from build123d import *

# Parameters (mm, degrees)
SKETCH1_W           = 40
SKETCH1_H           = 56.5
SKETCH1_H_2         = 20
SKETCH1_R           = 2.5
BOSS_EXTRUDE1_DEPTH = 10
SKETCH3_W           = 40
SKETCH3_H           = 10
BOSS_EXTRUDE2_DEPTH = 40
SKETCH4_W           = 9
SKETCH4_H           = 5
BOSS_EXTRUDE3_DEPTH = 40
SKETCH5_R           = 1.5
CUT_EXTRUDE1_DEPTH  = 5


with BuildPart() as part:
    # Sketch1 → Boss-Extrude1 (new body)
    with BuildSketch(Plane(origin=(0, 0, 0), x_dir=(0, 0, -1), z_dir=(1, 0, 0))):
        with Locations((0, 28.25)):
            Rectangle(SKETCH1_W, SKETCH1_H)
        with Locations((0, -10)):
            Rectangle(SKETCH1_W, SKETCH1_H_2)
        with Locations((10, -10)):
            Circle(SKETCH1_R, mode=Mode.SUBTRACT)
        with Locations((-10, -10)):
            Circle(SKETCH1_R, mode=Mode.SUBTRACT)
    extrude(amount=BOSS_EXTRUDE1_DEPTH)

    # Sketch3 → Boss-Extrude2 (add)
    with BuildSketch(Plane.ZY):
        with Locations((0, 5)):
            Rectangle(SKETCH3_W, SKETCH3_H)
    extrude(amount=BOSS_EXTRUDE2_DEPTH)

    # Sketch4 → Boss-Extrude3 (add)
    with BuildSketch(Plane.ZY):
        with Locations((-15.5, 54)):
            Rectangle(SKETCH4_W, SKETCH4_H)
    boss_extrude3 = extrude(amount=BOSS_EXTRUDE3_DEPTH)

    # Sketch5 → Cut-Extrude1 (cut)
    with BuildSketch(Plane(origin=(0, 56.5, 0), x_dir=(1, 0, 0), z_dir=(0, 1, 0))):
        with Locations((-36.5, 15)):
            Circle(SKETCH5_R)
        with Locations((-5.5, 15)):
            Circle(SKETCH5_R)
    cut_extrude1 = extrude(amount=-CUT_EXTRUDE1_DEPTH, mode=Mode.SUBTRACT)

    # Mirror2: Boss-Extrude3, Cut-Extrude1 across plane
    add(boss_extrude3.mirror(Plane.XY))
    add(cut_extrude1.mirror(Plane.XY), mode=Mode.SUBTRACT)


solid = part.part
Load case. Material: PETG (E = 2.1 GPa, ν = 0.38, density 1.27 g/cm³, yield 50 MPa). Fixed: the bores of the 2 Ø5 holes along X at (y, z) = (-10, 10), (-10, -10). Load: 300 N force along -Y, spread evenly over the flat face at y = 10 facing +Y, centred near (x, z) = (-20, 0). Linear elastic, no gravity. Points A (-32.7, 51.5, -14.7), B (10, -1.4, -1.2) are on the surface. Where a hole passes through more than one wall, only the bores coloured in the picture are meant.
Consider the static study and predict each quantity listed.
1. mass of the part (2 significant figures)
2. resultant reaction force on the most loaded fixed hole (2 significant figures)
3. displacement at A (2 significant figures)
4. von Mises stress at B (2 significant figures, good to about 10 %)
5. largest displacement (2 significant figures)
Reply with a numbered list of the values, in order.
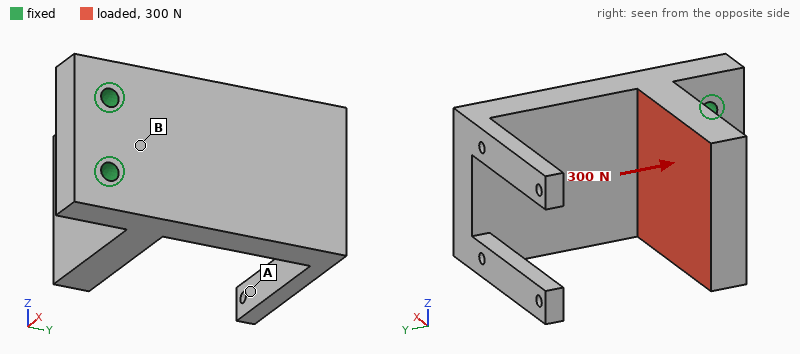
1. 63 g
2. 160 N
3. 0.96 mm
4. 8.4 MPa
5. 1.1 mm
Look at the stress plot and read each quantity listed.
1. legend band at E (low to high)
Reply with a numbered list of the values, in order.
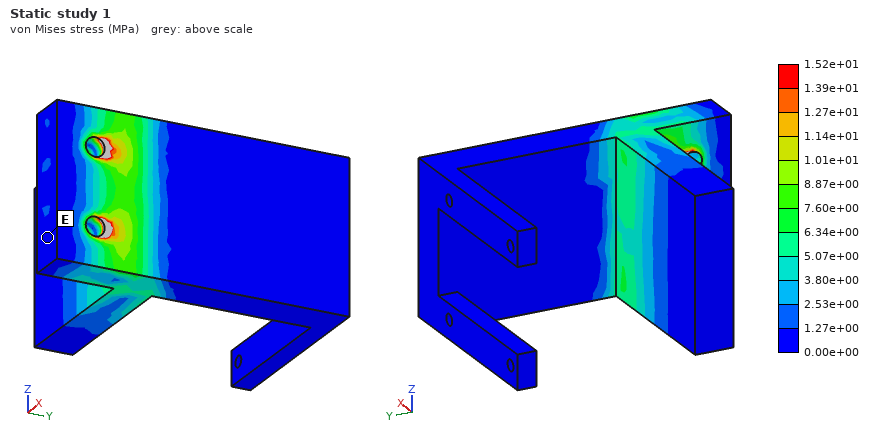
1. 0.00e+00 to 1.27e+00 MPa
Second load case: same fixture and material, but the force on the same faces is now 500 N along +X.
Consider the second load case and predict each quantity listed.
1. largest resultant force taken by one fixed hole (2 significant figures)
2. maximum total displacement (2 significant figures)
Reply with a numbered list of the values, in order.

1. 250 N
2. 1.0 mm
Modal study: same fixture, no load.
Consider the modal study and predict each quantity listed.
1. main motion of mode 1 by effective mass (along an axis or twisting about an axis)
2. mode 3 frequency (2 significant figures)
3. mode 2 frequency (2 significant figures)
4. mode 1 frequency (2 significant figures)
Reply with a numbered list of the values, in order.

1. along X
2. 560 Hz
3. 540 Hz
4. 350 Hz
